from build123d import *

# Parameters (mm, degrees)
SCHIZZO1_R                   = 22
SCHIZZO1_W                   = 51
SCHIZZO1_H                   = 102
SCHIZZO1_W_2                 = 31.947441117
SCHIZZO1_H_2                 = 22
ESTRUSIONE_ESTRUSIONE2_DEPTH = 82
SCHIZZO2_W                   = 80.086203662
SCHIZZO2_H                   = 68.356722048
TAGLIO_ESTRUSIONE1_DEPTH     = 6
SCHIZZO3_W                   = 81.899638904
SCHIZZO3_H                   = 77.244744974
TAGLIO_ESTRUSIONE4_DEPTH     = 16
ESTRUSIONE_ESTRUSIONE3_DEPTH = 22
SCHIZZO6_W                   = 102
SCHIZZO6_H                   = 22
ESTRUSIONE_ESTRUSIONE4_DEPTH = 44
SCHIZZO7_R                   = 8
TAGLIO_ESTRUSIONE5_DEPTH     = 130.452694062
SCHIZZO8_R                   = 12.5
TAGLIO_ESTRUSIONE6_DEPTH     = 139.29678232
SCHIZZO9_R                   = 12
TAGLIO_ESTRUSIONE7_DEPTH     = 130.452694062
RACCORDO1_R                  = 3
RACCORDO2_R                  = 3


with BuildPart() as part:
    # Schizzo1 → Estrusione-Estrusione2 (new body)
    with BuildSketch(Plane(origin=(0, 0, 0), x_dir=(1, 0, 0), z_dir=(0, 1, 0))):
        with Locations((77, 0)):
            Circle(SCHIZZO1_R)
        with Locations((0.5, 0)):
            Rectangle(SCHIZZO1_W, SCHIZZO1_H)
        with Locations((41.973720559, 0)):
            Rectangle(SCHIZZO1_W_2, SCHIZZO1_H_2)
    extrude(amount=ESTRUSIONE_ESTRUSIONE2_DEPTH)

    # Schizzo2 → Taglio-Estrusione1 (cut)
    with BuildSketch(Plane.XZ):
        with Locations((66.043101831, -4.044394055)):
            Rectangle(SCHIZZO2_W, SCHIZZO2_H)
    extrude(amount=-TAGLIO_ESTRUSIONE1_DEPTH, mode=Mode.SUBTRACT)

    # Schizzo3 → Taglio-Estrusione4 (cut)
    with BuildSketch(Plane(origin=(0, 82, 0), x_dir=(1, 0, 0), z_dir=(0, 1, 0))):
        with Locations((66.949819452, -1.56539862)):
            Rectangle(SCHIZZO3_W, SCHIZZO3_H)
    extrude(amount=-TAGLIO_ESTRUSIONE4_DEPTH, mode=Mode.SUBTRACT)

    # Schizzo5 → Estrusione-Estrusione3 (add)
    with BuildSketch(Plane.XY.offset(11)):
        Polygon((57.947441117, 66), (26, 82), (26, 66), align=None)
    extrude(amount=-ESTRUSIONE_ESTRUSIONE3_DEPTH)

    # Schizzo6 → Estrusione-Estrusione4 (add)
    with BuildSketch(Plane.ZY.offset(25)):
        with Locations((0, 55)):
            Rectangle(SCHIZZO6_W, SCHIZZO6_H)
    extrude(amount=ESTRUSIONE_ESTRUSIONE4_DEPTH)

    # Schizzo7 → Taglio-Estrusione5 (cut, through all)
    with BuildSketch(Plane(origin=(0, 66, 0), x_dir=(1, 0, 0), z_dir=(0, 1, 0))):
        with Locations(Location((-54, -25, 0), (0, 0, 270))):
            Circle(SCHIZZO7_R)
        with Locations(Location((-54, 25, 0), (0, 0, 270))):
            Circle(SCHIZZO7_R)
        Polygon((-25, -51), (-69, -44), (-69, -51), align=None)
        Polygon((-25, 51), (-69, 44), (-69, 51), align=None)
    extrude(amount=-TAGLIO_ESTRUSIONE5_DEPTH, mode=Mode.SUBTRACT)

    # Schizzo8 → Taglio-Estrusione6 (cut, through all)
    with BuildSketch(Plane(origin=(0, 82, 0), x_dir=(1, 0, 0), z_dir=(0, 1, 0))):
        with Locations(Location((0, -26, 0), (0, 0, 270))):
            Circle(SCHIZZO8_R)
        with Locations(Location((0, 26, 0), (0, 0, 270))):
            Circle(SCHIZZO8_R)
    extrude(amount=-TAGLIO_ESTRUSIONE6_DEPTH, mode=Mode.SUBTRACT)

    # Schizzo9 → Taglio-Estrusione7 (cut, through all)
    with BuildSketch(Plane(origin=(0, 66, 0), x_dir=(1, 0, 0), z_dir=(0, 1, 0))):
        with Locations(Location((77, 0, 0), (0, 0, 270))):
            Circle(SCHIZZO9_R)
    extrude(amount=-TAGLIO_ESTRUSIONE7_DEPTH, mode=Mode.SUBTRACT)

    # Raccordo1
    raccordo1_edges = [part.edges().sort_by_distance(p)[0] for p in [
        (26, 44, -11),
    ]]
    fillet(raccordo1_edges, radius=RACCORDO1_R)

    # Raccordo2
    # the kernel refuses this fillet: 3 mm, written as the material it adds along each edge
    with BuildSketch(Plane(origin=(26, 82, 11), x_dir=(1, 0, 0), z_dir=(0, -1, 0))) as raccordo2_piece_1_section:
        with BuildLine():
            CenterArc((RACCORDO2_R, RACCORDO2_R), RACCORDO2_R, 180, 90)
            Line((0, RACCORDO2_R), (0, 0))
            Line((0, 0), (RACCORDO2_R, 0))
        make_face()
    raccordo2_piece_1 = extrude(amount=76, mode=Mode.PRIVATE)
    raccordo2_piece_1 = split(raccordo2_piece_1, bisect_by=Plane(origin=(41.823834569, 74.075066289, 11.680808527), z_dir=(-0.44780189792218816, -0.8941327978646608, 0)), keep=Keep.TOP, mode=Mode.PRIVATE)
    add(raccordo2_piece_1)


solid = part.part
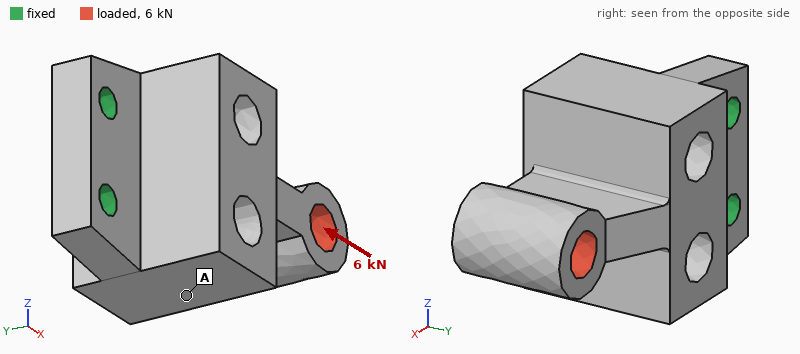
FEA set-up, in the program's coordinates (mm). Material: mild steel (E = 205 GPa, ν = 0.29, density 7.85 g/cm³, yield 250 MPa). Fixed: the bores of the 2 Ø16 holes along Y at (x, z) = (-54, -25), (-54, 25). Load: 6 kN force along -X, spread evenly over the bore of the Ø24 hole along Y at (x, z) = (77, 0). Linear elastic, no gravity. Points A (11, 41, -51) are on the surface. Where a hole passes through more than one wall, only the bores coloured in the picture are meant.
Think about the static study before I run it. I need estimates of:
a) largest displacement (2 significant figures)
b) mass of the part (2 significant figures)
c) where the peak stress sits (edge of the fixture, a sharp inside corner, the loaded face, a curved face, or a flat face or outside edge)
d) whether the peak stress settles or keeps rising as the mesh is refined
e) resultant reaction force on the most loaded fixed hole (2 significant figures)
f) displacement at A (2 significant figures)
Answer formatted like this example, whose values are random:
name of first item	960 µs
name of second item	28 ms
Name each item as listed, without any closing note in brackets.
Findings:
largest displacement	34 µm
mass of the part	4.2 kg
where the peak stress sits	edge of the fixture
whether the peak stress settles or keeps rising as the mesh is refined	keeps rising
resultant reaction force on the most loaded fixed hole	3.0 kN
displacement at A	11 µm
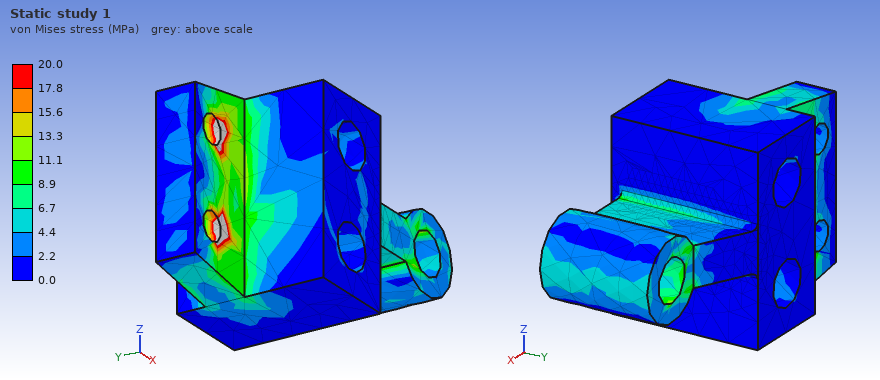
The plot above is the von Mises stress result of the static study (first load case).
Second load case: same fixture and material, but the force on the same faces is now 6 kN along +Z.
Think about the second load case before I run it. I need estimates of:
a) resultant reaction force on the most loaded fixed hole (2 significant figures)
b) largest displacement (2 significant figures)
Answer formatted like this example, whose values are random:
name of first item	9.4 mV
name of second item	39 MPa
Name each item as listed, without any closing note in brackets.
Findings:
resultant reaction force on the most loaded fixed hole	13 kN
largest displacement	83 µm
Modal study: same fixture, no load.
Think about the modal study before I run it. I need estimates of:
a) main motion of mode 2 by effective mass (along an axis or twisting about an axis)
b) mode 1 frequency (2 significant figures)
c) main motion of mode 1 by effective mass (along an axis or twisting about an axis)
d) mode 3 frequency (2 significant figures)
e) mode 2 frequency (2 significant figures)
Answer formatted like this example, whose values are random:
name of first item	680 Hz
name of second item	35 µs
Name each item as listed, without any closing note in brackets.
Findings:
main motion of mode 2 by effective mass	along Z
mode 1 frequency	900 Hz
main motion of mode 1 by effective mass	along Y
mode 3 frequency	3200 Hz
mode 2 frequency	2000 Hz
